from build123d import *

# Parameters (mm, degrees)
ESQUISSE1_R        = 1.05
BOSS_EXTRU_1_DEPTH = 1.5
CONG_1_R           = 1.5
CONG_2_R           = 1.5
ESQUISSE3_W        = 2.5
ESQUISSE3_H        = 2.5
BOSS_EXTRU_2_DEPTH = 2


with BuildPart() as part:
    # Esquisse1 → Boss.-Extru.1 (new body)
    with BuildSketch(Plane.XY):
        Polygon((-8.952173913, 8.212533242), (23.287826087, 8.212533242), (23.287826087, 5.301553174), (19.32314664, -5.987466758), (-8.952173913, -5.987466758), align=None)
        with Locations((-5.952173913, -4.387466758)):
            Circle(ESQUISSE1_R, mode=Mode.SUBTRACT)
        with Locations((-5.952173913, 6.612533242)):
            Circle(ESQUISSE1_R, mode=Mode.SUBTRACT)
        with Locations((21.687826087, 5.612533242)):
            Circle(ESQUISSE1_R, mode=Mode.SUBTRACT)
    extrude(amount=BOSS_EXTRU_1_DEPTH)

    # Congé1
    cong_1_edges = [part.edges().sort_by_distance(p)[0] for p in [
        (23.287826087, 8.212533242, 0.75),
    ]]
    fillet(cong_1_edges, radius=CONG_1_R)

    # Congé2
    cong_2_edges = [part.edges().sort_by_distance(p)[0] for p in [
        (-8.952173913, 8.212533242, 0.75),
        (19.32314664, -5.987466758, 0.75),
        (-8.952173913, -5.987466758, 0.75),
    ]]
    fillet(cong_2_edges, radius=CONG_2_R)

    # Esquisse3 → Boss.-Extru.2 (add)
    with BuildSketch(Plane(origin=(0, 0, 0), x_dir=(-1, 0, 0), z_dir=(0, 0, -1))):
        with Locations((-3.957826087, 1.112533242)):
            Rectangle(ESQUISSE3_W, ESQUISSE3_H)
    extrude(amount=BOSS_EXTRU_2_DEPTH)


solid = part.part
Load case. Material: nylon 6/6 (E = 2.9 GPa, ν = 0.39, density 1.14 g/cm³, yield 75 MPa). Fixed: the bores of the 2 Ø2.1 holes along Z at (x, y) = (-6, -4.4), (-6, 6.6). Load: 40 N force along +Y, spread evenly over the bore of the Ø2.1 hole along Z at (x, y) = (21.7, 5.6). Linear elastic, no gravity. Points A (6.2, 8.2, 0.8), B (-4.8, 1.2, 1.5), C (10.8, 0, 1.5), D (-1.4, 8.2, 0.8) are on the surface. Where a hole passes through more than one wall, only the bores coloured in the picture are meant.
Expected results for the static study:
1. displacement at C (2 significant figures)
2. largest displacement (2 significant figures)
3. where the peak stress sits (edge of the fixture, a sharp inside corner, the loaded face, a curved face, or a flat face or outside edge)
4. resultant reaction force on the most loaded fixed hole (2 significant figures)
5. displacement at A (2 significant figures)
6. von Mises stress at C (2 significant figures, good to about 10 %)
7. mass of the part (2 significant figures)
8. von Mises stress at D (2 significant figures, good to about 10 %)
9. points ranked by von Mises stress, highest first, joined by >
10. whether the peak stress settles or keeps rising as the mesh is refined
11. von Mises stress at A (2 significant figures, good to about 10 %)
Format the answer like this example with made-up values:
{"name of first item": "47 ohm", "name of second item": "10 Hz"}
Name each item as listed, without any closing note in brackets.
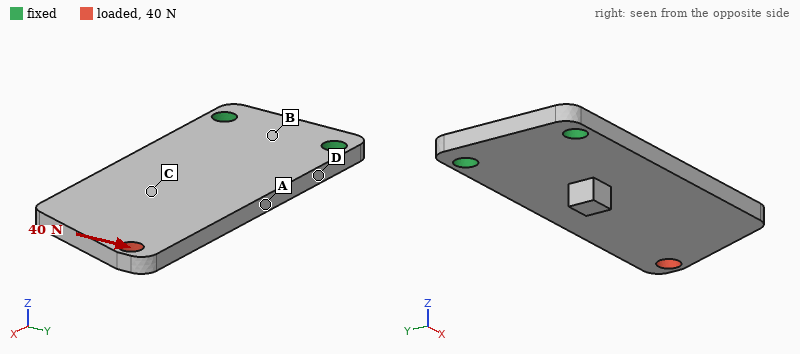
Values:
{"displacement at C": "0.14 mm", "largest displacement": "0.37 mm", "where the peak stress sits": "edge of the fixture", "resultant reaction force on the most loaded fixed hole": "98 N", "displacement at A": "0.11 mm", "von Mises stress at C": "5.3 MPa", "mass of the part": "0.74 g", "von Mises stress at D": "18 MPa", "points ranked by von Mises stress, highest first, joined by >": "D > A > C > B", "whether the peak stress settles or keeps rising as the mesh is refined": "keeps rising", "von Mises stress at A": "12 MPa"}
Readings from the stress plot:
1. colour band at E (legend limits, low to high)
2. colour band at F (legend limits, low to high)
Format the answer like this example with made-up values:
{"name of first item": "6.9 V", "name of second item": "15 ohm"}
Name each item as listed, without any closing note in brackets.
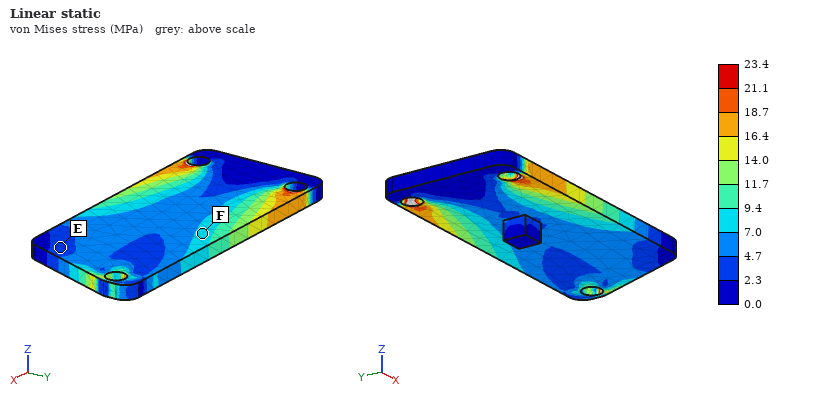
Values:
{"colour band at E": "2.3 to 4.7 MPa", "colour band at F": "7.0 to 9.4 MPa"}
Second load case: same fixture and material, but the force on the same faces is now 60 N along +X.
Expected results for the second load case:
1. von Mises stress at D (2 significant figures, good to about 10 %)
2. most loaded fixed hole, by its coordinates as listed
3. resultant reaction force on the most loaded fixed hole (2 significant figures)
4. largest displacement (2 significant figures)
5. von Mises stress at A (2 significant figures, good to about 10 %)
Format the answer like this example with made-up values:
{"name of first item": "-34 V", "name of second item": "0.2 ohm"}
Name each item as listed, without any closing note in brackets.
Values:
{"von Mises stress at D": "8.7 MPa", "most loaded fixed hole, by its coordinates as listed": "(-6, 6.6)", "resultant reaction force on the most loaded fixed hole": "54 N", "largest displacement": "0.14 mm", "von Mises stress at A": "8.2 MPa"}
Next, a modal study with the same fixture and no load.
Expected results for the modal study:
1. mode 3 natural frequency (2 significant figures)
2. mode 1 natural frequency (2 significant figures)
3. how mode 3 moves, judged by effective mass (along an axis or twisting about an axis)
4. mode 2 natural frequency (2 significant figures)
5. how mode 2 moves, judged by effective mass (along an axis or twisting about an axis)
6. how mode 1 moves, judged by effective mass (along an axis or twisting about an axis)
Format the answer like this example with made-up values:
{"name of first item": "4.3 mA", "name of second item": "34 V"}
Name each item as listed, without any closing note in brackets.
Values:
{"mode 3 natural frequency": "3200 Hz", "mode 1 natural frequency": "530 Hz", "how mode 3 moves, judged by effective mass": "along Z", "mode 2 natural frequency": "2200 Hz", "how mode 2 moves, judged by effective mass": "twisting about X", "how mode 1 moves, judged by effective mass": "along Z"}
